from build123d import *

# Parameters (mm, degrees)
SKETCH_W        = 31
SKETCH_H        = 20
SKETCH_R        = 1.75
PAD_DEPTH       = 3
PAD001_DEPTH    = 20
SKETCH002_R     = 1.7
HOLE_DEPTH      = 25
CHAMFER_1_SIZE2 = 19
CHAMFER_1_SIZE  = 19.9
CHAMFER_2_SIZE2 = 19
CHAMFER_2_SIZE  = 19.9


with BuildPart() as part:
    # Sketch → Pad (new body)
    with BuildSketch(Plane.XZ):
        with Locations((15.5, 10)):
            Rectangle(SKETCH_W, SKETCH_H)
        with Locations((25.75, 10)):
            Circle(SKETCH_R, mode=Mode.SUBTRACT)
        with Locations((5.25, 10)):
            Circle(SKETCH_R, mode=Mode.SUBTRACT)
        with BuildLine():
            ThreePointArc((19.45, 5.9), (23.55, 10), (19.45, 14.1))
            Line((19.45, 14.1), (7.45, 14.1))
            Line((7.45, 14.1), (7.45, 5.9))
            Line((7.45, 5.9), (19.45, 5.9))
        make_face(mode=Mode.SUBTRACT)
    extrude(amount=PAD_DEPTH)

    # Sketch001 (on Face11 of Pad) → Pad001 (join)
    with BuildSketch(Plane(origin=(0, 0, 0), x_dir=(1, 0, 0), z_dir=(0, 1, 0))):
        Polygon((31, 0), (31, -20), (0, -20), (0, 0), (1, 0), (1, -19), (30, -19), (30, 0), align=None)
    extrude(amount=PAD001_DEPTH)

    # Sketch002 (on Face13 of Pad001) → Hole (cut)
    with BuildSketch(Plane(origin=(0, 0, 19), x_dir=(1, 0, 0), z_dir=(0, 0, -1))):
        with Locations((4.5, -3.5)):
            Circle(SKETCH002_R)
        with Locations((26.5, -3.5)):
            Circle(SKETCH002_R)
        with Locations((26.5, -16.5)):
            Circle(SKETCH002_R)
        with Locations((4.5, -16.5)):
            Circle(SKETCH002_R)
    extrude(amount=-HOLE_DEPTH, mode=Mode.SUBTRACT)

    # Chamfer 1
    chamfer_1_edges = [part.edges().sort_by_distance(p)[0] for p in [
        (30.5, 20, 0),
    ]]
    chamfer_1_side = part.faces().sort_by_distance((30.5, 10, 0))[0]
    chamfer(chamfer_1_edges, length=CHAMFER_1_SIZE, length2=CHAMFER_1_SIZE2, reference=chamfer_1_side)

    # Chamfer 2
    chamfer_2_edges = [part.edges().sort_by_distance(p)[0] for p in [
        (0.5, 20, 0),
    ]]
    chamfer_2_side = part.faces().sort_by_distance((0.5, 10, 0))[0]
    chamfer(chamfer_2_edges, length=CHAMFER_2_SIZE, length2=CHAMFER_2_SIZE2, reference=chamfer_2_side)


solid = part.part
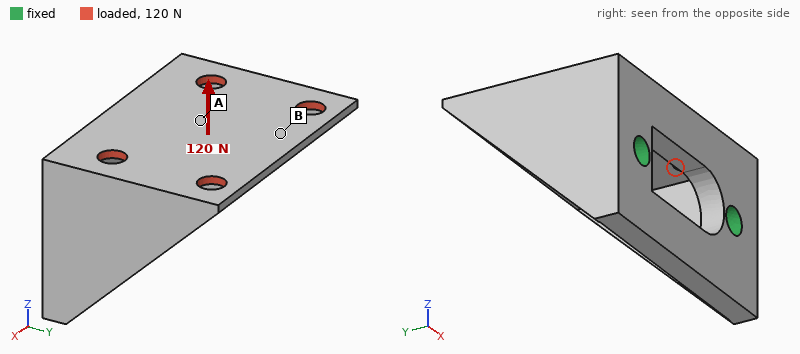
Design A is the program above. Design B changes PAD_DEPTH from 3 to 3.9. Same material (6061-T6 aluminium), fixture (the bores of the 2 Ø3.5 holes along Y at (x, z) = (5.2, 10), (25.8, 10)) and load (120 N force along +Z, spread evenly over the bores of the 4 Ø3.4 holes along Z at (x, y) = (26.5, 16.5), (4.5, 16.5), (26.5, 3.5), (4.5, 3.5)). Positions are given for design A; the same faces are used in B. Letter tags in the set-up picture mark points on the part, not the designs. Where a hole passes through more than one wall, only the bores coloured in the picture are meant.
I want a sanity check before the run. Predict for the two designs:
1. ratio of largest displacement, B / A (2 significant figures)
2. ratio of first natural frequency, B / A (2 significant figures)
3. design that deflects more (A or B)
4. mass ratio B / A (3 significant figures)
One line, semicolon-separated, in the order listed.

0.91; 1.0; A; 1.18
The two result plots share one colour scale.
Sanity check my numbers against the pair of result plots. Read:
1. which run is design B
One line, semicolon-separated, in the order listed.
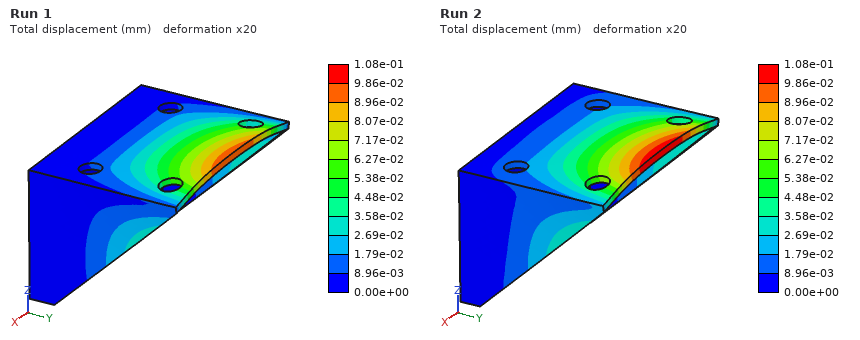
Run 1
